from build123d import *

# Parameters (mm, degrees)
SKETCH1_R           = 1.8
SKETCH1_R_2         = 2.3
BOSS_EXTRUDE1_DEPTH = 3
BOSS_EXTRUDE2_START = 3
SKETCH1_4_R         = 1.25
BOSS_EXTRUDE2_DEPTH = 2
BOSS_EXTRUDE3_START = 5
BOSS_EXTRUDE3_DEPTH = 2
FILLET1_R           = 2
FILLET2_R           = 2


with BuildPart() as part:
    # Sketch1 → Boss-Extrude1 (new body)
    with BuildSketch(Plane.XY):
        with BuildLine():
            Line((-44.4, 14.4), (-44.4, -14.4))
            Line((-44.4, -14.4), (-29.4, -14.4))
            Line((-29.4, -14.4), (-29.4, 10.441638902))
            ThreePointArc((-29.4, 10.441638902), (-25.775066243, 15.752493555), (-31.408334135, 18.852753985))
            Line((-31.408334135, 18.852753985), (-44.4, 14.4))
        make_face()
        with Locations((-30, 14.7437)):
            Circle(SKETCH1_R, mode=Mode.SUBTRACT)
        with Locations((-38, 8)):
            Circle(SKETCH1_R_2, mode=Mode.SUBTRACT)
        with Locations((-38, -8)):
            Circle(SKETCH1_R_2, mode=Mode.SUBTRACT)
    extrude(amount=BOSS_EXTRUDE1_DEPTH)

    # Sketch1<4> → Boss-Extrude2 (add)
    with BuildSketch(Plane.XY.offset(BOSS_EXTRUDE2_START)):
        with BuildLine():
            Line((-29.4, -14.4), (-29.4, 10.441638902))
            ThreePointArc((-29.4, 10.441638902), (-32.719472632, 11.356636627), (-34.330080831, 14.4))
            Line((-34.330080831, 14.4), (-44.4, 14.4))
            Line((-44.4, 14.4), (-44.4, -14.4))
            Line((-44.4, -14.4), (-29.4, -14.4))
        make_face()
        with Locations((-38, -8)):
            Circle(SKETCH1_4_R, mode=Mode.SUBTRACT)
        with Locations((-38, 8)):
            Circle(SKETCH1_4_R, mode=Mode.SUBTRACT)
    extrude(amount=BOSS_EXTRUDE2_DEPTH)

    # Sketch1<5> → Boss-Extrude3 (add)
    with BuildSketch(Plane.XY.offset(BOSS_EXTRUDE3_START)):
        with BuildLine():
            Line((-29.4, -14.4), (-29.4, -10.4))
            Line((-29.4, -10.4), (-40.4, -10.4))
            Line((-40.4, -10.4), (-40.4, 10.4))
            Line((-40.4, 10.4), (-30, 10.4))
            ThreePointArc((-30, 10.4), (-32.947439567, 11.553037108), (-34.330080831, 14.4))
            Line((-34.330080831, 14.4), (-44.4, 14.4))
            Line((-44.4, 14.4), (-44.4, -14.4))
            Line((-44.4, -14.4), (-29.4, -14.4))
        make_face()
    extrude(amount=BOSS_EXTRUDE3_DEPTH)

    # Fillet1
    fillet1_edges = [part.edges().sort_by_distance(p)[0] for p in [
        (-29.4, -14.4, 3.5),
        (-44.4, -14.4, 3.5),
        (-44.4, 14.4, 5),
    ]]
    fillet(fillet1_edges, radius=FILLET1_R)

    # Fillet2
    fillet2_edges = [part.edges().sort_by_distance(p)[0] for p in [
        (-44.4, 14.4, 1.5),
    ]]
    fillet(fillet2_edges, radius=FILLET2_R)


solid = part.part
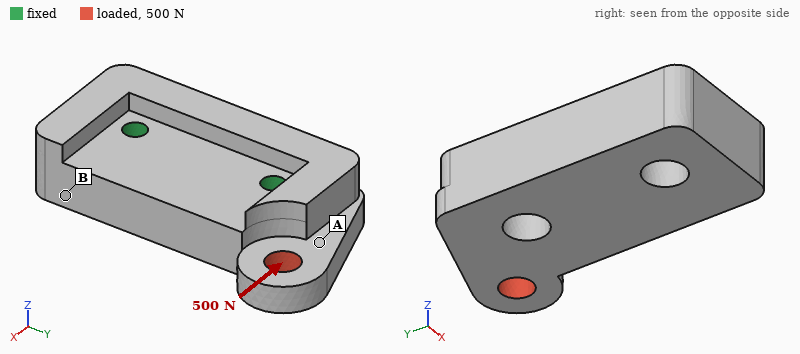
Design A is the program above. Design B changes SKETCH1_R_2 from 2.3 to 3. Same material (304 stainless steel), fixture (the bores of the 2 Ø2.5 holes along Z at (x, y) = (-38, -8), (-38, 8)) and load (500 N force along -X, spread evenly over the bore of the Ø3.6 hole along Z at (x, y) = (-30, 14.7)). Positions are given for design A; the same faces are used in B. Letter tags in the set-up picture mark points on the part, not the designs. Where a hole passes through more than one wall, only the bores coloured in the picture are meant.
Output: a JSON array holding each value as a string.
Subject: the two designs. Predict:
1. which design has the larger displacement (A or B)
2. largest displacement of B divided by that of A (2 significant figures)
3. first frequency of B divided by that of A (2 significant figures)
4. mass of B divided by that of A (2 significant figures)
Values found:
["B", "1.1", "0.97", "0.97"]
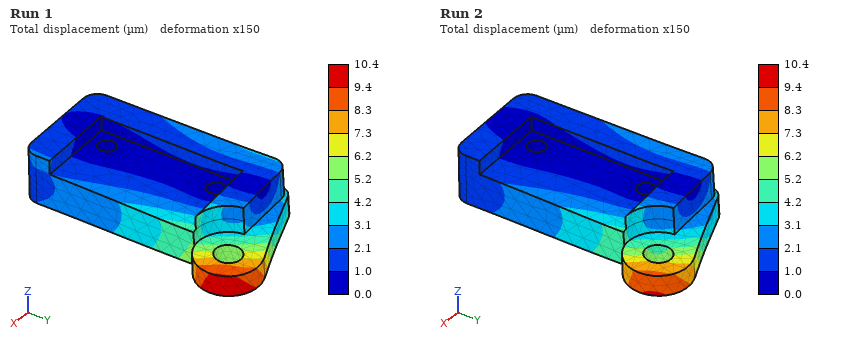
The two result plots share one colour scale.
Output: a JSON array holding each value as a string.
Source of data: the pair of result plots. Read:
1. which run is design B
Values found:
["Run 1"]
